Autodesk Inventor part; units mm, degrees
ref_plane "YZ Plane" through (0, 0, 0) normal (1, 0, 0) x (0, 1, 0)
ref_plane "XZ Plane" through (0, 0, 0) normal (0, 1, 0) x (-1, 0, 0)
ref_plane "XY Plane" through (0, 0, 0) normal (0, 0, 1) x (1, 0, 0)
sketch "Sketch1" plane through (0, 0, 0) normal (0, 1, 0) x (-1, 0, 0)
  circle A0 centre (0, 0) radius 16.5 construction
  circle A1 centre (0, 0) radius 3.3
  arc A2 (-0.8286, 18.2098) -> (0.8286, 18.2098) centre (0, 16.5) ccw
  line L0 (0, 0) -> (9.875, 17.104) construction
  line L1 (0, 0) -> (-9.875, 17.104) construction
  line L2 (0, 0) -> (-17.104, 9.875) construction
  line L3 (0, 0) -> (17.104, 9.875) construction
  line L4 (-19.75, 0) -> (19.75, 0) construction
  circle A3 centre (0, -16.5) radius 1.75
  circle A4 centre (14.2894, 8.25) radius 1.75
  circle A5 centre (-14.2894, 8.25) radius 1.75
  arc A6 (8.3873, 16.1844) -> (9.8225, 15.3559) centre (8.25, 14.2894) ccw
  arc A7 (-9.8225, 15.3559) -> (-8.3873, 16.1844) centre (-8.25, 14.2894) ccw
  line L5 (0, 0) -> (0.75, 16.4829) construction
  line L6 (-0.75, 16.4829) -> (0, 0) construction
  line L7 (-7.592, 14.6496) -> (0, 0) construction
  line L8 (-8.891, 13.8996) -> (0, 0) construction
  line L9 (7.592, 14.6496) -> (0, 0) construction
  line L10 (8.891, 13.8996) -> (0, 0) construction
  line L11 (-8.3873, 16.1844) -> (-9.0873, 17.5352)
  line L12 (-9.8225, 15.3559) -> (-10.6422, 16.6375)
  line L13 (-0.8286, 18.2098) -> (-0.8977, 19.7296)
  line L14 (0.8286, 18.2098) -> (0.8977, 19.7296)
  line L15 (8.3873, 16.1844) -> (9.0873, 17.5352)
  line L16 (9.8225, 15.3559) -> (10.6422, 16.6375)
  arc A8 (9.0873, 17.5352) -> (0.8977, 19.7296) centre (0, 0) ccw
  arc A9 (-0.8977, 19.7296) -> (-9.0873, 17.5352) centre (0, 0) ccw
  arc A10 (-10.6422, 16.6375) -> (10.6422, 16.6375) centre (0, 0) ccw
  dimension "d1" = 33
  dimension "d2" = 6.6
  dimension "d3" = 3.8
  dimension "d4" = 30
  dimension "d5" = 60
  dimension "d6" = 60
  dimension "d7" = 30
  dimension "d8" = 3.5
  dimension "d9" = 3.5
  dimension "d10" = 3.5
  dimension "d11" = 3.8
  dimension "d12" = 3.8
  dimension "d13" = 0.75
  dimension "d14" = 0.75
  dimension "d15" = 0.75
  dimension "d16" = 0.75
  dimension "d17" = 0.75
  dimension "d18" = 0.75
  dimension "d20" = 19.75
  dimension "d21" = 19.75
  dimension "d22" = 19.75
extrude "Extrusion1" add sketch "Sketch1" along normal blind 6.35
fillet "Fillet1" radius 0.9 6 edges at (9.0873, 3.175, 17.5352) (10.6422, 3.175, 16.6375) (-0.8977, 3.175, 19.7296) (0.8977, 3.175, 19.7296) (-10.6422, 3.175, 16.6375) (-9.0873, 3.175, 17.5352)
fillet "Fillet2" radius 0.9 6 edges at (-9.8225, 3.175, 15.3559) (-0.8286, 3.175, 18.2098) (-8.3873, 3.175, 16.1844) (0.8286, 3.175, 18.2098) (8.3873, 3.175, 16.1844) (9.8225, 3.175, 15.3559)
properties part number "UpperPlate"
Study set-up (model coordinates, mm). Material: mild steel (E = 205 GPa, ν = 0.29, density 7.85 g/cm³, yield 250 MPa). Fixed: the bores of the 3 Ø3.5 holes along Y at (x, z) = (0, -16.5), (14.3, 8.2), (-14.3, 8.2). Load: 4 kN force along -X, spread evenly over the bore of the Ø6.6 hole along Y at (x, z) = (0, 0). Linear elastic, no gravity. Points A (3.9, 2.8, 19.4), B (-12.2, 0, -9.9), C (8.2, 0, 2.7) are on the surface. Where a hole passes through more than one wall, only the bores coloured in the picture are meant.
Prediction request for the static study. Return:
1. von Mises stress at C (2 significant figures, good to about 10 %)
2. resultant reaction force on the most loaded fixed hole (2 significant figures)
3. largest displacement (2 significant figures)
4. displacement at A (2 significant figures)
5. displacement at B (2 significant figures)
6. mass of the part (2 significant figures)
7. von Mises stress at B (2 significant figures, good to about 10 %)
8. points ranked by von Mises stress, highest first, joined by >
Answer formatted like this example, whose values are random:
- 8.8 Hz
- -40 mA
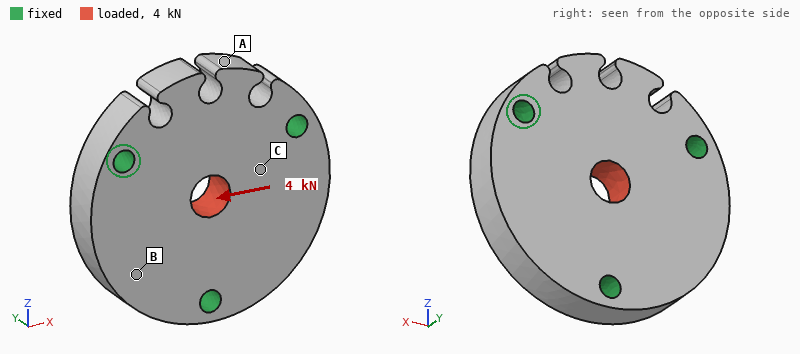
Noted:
- 26 MPa
- 1.4 kN
- 2.3 µm
- 0.45 µm
- 1.2 µm
- 56 g
- 10 MPa
- C > B > A
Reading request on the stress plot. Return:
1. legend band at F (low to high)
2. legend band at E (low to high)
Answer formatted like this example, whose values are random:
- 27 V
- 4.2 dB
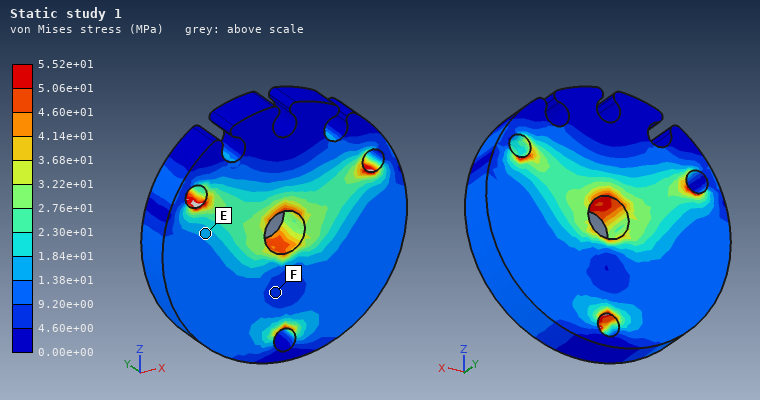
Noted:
- 4.60e+00 to 9.20e+00 MPa
- 1.38e+01 to 1.84e+01 MPa
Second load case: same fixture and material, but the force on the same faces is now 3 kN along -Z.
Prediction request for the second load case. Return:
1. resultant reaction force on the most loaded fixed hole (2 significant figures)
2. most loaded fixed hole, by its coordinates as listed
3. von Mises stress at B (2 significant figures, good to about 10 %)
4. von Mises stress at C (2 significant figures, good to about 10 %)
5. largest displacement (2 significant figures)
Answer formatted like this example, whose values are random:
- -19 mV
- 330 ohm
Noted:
- 1.2 kN
- (0, -16.5)
- 4.5 MPa
- 11 MPa
- 2.1 µm
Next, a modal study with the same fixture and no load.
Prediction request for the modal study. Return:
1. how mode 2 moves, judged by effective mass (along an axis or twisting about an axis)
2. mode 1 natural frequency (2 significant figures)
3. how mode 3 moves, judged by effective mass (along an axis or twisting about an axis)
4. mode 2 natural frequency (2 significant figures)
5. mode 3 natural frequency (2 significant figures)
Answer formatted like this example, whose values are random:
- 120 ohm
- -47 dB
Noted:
- twisting about Z
- 22 kHz
- along Y
- 24 kHz
- 26 kHz
